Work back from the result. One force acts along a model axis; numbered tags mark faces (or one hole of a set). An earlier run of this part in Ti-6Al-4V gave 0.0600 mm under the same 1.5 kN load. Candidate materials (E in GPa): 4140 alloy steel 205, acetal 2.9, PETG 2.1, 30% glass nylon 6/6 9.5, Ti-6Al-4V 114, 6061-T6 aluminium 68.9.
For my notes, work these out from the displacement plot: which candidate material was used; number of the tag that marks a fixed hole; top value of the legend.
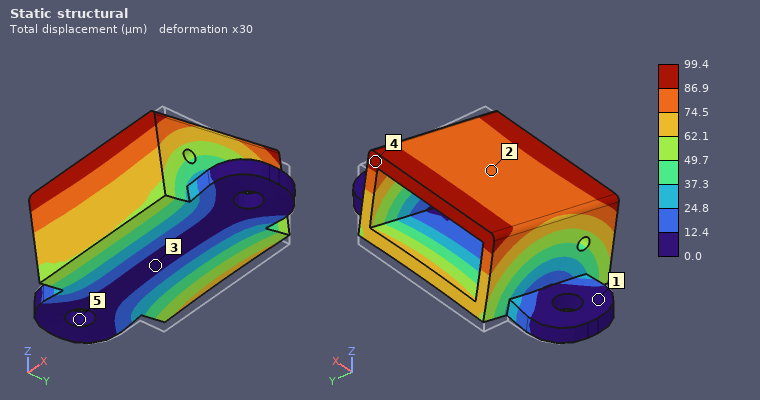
6061-T6 aluminium
5
99.4 µm
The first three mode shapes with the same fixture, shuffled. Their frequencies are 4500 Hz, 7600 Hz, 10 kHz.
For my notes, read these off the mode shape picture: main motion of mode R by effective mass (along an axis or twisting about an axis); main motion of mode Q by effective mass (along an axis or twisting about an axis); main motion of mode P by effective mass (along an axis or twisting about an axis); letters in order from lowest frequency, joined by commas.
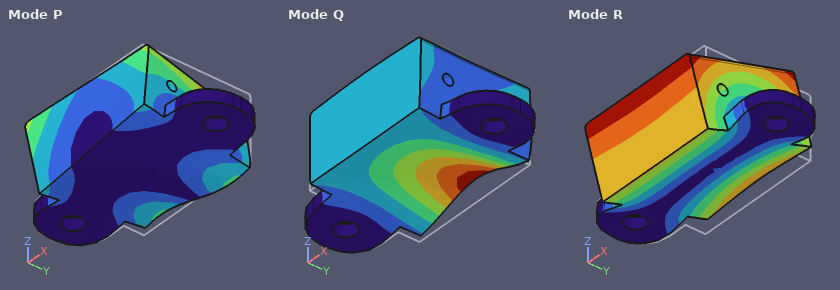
along Y
along Z
along X
R, P, Q
